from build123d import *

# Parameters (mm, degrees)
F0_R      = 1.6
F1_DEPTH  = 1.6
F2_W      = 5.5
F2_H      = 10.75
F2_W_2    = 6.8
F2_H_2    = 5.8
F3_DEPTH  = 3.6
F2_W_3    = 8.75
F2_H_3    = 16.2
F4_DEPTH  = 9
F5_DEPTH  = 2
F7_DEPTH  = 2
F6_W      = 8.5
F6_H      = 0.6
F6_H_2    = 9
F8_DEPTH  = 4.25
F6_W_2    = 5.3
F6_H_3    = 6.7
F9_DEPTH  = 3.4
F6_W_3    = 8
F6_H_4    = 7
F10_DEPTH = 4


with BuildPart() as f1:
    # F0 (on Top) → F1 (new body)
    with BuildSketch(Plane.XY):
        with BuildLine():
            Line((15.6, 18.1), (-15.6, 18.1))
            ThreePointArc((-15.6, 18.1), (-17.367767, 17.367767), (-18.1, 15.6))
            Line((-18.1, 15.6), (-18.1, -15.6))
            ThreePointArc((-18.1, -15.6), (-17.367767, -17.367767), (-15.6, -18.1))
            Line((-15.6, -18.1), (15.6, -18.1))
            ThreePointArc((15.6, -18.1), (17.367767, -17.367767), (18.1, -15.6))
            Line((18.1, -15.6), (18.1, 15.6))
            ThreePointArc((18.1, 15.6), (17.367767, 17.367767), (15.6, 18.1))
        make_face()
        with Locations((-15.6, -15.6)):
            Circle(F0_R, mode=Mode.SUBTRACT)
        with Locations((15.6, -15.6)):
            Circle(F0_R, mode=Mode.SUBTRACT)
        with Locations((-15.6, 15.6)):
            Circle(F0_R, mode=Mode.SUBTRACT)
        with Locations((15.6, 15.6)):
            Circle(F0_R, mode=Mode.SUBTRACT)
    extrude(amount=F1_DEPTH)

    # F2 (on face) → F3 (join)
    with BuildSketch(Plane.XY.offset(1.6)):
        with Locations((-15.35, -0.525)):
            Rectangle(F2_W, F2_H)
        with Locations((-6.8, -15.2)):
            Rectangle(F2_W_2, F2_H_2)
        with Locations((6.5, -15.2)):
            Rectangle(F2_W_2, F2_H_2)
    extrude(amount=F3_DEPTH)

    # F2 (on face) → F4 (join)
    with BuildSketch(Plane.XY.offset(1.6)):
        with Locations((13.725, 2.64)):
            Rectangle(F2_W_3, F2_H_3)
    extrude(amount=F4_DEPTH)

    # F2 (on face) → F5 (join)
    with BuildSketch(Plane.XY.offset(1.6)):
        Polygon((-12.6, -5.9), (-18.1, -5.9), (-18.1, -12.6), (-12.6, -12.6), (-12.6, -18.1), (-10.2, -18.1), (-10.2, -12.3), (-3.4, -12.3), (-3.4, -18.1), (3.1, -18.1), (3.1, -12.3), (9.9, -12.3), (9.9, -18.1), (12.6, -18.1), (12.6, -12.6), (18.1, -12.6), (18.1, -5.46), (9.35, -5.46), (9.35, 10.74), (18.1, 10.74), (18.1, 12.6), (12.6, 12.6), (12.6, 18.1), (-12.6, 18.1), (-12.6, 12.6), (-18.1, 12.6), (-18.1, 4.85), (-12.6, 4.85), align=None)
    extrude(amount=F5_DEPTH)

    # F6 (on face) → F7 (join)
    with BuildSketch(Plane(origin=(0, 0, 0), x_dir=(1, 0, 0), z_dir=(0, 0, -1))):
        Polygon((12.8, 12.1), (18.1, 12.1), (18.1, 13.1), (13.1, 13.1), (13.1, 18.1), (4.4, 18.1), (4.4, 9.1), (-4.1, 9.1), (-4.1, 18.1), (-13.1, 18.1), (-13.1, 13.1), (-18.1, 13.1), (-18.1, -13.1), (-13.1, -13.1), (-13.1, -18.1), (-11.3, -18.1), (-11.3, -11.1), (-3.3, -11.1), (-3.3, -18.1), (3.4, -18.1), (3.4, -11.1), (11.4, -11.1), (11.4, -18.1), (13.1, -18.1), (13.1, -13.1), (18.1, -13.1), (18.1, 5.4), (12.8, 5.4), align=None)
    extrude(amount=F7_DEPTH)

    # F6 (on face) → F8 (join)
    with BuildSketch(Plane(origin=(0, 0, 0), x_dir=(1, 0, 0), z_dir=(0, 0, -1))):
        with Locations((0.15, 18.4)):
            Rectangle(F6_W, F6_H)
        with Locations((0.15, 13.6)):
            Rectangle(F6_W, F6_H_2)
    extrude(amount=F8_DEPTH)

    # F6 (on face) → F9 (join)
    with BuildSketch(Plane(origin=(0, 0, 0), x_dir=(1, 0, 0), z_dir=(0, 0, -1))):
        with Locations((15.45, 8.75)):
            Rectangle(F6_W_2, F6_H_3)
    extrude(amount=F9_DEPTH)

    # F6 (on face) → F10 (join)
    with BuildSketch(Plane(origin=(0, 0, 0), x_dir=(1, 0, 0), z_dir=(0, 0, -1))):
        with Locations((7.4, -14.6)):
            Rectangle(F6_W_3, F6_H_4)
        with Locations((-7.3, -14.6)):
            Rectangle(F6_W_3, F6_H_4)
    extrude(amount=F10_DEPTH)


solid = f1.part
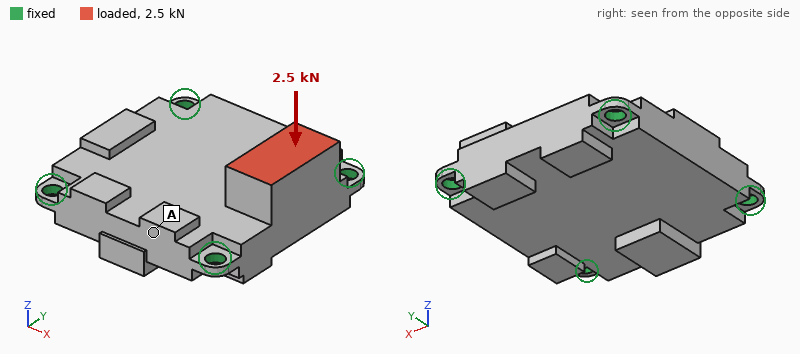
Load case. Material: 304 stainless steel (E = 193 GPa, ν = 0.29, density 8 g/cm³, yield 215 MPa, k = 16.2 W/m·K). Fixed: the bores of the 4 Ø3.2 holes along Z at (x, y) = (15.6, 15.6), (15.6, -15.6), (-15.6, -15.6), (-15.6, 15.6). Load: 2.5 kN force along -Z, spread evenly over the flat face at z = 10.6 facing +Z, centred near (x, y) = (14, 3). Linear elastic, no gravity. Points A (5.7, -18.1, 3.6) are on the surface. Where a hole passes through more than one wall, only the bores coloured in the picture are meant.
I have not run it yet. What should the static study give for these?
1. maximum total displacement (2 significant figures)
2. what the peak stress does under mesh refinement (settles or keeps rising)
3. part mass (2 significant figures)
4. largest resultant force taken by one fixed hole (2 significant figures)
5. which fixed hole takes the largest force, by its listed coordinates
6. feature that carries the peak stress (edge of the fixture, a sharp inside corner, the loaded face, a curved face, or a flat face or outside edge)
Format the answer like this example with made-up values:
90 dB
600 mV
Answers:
17 µm
keeps rising
68 g
1.4 kN
(15.6, 15.6)
edge of the fixture
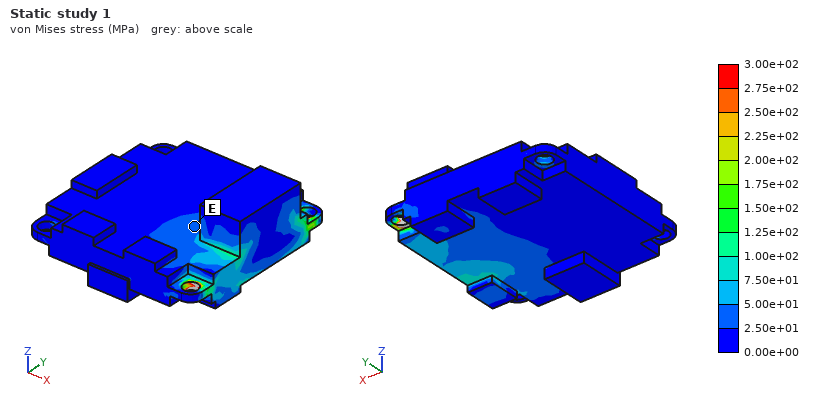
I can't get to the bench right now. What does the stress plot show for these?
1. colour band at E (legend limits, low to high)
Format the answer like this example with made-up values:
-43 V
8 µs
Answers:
2.50e+01 to 5.00e+01 MPa
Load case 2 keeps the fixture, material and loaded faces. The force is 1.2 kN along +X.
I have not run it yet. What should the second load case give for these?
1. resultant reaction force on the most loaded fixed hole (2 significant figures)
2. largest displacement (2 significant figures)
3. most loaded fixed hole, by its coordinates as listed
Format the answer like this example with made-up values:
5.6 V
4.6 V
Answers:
480 N
15 µm
(15.6, 15.6)
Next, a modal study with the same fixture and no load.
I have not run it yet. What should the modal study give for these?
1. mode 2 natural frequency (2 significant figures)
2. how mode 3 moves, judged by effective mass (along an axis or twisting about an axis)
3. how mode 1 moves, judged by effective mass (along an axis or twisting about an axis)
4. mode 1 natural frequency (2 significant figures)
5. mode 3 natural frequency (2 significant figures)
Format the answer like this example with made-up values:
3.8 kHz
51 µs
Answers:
17 kHz
twisting about X
along Z
12 kHz
19 kHz
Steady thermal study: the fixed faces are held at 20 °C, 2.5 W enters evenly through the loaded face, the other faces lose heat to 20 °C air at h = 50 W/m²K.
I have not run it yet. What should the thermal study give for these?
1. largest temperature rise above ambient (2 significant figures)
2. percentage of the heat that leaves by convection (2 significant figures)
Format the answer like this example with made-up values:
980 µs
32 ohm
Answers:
19 K
41 %
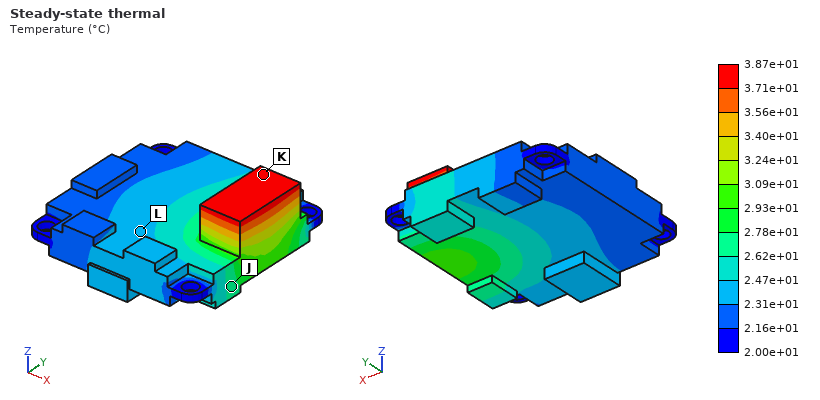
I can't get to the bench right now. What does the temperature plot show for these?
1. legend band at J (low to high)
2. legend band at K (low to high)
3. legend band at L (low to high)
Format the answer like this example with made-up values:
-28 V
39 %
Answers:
2.62e+01 to 2.78e+01 °C
3.71e+01 to 3.87e+01 °C
2.31e+01 to 2.47e+01 °C
